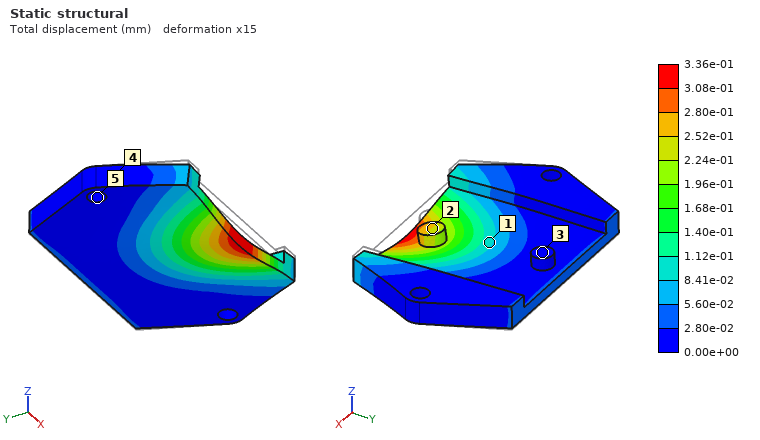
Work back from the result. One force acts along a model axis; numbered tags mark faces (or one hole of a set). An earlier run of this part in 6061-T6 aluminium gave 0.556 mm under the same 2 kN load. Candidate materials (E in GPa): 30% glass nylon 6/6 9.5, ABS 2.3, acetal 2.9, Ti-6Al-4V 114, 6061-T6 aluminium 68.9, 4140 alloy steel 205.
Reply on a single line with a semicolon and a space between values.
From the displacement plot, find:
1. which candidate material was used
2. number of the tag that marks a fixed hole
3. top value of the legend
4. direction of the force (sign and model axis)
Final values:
Ti-6Al-4V; 5; 3.36e-01 mm; -Z
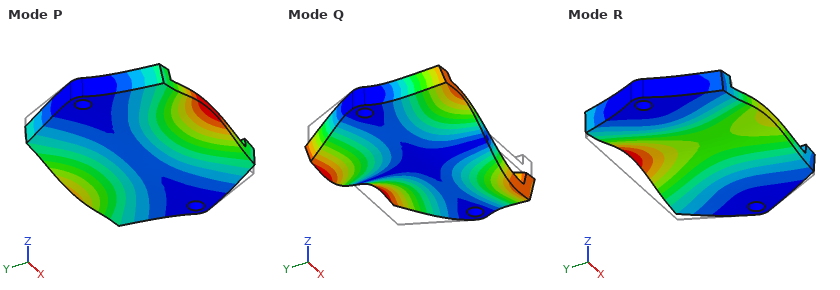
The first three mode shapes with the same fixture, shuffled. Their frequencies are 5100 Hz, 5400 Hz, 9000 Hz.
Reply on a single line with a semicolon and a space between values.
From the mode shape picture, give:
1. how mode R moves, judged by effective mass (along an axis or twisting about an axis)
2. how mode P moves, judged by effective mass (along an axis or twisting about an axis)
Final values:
along Z; twisting about X
